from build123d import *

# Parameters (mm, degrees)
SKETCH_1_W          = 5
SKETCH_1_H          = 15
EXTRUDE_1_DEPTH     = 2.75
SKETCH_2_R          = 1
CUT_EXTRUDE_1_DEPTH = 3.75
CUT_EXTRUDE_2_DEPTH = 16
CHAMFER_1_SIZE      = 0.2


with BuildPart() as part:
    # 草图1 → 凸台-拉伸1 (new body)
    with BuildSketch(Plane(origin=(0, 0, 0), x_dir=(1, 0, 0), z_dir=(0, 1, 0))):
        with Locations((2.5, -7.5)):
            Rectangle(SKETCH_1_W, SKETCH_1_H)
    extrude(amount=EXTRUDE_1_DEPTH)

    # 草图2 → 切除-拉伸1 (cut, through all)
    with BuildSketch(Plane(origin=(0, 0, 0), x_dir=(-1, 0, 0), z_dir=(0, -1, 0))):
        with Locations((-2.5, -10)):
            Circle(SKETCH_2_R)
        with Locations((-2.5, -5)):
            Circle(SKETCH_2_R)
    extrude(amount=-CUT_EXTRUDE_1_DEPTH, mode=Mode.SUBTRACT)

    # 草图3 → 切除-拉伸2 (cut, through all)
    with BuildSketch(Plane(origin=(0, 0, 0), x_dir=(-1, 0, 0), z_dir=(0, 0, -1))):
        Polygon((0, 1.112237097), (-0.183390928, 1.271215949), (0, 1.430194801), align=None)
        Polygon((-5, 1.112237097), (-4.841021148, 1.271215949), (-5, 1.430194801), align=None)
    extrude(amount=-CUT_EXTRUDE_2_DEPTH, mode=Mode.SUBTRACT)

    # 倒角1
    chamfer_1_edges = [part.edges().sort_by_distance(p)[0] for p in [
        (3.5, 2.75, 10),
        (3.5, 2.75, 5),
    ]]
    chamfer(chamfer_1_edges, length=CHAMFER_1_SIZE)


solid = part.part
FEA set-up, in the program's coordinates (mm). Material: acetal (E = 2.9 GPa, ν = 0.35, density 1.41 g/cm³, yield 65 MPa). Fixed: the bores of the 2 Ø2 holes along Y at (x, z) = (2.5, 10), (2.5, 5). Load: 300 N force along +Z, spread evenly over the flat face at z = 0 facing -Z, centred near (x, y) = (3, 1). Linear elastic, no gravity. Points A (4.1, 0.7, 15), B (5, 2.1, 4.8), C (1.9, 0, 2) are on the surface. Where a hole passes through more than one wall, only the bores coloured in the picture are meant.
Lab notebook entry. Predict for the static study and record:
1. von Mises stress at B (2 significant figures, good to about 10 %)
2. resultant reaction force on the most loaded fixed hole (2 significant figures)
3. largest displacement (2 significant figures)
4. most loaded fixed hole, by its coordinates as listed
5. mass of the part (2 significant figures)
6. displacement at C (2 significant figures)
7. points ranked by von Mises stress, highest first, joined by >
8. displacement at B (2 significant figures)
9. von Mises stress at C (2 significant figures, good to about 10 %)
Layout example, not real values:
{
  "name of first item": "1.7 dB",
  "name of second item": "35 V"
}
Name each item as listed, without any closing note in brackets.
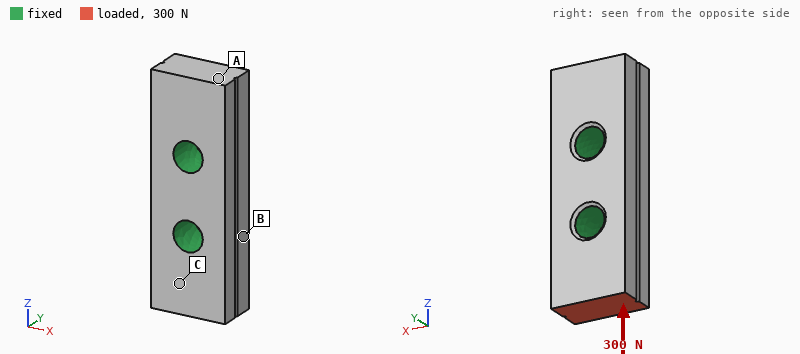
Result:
{
  "von Mises stress at B": "12 MPa",
  "resultant reaction force on the most loaded fixed hole": "280 N",
  "largest displacement": "40 µm",
  "most loaded fixed hole, by its coordinates as listed": "(2.5, 5)",
  "mass of the part": "0.26 g",
  "displacement at C": "21 µm",
  "points ranked by von Mises stress, highest first, joined by >": "C > B > A",
  "displacement at B": "10 µm",
  "von Mises stress at C": "25 MPa"
}
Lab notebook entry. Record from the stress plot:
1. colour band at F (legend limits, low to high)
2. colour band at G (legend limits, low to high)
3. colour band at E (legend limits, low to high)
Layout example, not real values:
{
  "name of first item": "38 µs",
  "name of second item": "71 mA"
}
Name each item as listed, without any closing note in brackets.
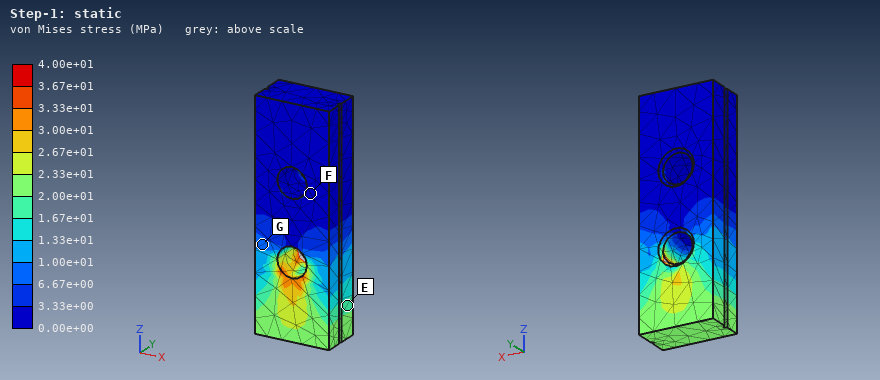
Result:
{
  "colour band at F": "0.00e+00 to 3.33e+00 MPa",
  "colour band at G": "6.67e+00 to 1.00e+01 MPa",
  "colour band at E": "1.67e+01 to 2.00e+01 MPa"
}
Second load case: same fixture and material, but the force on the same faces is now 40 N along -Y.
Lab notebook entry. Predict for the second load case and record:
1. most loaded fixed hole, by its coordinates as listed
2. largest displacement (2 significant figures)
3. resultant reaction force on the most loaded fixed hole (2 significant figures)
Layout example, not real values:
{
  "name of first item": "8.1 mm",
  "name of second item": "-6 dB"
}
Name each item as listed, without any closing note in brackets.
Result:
{
  "most loaded fixed hole, by its coordinates as listed": "(2.5, 5)",
  "largest displacement": "71 µm",
  "resultant reaction force on the most loaded fixed hole": "44 N"
}
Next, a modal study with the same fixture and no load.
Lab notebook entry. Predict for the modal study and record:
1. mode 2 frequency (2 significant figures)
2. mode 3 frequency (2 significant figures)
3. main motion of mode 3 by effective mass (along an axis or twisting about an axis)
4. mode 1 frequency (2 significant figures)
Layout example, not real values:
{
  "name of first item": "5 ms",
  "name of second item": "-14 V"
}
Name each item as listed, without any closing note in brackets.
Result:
{
  "mode 2 frequency": "25 kHz",
  "mode 3 frequency": "27 kHz",
  "main motion of mode 3 by effective mass": "twisting about Y",
  "mode 1 frequency": "24 kHz"
}
